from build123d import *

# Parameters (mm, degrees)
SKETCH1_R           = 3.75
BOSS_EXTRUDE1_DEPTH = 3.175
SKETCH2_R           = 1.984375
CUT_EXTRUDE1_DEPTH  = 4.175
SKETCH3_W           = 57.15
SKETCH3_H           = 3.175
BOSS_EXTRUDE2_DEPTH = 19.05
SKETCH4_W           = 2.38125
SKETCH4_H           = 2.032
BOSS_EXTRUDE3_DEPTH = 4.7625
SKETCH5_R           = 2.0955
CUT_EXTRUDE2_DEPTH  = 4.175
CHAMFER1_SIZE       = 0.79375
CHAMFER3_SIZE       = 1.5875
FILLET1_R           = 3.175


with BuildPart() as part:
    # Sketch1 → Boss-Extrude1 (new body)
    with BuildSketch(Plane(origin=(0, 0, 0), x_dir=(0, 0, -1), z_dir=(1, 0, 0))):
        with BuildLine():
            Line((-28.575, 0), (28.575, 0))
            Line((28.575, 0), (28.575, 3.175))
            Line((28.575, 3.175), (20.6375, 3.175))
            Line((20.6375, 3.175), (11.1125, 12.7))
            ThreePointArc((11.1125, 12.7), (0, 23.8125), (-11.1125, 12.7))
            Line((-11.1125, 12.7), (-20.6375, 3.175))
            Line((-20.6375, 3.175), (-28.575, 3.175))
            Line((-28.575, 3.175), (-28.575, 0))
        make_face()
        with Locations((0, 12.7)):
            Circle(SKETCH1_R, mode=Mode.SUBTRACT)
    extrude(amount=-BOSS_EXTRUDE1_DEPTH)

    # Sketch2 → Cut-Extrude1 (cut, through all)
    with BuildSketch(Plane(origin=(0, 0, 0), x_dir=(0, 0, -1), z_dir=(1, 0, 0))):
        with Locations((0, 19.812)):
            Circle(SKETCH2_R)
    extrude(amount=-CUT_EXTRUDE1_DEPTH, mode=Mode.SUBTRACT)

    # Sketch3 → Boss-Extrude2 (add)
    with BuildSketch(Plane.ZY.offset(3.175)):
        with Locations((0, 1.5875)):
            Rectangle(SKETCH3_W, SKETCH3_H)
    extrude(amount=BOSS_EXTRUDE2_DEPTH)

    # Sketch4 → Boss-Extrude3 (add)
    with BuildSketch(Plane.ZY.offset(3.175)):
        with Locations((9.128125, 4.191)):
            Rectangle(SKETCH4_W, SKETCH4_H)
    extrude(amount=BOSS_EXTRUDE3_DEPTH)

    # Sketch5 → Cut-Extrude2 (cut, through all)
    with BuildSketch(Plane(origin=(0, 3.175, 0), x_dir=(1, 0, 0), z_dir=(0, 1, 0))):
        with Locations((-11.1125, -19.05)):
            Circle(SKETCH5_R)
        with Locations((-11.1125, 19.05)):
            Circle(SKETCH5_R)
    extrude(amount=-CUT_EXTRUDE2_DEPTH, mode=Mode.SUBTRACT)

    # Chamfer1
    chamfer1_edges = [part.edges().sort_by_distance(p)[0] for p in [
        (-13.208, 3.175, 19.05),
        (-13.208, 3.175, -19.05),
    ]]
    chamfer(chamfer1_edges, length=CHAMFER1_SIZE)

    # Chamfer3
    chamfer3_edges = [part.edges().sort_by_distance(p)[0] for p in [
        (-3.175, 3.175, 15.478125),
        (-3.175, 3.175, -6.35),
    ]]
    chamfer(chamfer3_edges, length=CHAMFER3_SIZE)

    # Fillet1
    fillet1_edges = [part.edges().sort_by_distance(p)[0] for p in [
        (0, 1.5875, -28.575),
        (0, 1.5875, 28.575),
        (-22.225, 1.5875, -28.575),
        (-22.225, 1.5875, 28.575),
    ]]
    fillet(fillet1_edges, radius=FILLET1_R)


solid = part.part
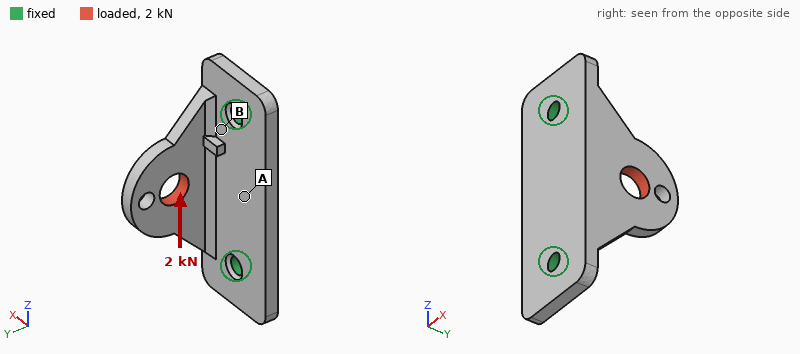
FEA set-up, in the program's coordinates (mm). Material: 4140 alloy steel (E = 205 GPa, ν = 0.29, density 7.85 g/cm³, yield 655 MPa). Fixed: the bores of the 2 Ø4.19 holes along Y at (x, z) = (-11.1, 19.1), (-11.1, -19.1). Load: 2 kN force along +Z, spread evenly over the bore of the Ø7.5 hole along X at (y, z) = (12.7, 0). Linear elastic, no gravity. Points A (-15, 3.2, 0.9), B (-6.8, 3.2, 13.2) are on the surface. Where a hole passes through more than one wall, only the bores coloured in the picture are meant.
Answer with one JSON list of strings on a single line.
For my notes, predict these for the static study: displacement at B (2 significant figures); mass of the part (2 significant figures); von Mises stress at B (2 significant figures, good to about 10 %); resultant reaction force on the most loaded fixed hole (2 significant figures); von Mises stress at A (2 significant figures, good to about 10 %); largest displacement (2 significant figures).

["4.4 µm", "42 g", "76 MPa", "1.3 kN", "21 MPa", "24 µm"]
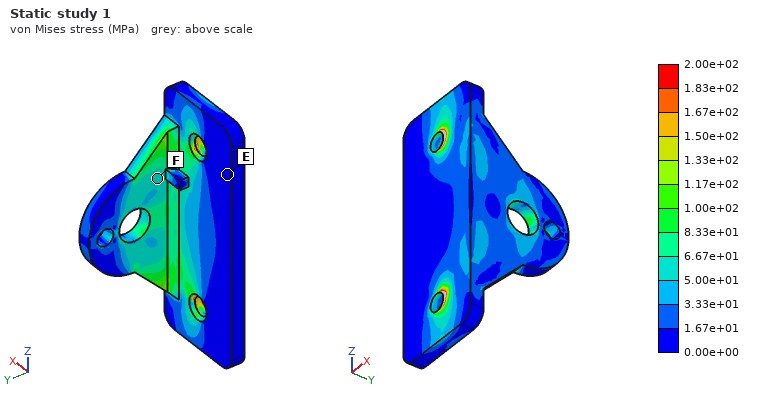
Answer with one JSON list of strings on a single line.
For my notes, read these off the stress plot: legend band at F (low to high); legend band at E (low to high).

["5.00e+01 to 6.67e+01 MPa", "0.00e+00 to 1.67e+01 MPa"]
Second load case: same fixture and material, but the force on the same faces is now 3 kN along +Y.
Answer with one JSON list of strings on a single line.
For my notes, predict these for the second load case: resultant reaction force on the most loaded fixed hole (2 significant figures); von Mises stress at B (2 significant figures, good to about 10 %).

["1.7 kN", "160 MPa"]
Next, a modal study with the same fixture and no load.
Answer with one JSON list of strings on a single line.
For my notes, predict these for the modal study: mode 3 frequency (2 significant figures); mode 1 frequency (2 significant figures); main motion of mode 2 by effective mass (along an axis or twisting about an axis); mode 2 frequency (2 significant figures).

["12 kHz", "5000 Hz", "along Y", "11 kHz"]
